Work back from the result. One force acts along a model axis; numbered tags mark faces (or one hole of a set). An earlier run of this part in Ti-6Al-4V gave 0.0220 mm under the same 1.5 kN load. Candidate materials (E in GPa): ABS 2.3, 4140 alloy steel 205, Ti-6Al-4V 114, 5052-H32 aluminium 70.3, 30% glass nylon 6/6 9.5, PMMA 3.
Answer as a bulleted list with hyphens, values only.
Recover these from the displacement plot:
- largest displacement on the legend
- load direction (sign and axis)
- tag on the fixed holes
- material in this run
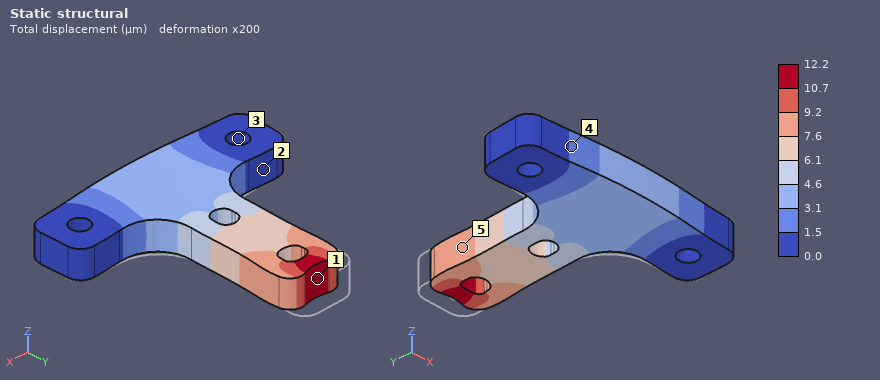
- 12.2 µm
- -Y
- 3
- 4140 alloy steel
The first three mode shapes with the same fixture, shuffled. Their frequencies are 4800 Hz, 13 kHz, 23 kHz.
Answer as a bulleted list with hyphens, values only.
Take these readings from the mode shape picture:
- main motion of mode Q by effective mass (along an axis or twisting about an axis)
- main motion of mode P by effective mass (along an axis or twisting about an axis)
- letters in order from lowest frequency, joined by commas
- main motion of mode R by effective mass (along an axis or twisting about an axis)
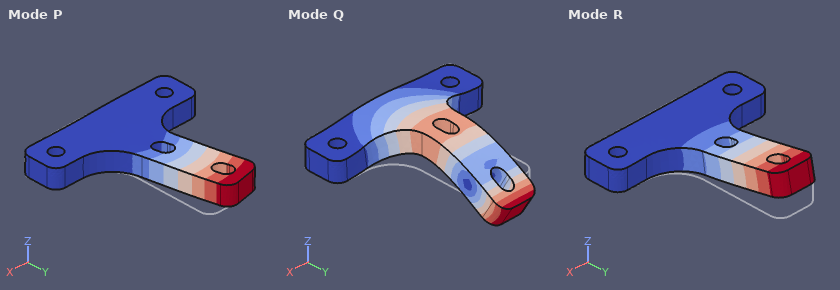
- along Z
- along X
- R, P, Q
- along Z
